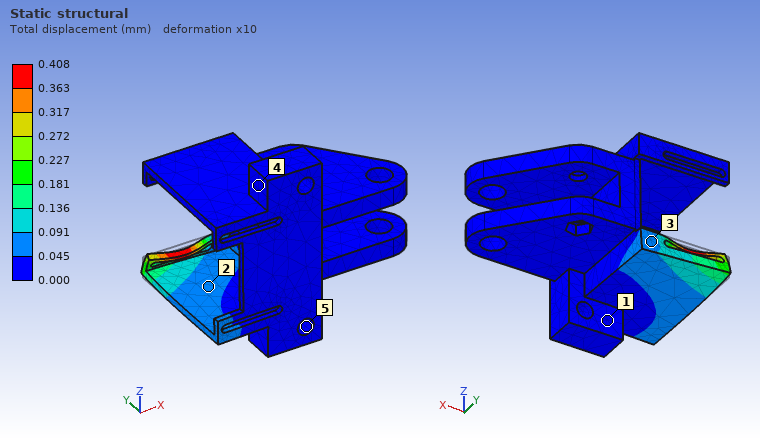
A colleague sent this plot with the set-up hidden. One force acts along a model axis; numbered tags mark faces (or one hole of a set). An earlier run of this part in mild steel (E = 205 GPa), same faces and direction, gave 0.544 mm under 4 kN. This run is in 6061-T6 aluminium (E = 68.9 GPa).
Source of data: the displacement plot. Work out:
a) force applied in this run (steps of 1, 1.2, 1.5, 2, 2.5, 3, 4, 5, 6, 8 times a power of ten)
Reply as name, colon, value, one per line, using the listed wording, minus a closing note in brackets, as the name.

force applied in this run: 1 kN
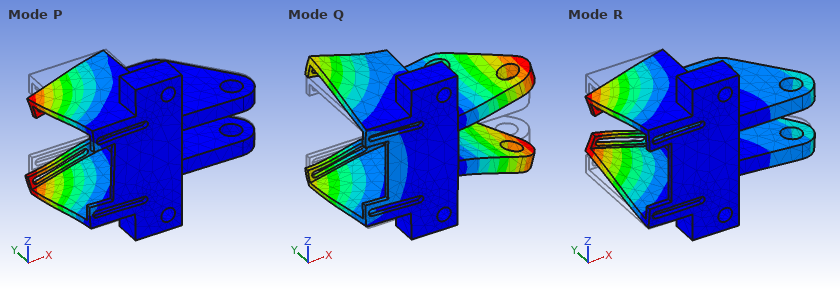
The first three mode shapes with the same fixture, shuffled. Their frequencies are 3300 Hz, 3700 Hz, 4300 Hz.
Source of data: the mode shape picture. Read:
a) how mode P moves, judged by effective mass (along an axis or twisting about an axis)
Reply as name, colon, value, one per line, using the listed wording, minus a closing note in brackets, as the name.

how mode P moves, judged by effective mass: along Z
